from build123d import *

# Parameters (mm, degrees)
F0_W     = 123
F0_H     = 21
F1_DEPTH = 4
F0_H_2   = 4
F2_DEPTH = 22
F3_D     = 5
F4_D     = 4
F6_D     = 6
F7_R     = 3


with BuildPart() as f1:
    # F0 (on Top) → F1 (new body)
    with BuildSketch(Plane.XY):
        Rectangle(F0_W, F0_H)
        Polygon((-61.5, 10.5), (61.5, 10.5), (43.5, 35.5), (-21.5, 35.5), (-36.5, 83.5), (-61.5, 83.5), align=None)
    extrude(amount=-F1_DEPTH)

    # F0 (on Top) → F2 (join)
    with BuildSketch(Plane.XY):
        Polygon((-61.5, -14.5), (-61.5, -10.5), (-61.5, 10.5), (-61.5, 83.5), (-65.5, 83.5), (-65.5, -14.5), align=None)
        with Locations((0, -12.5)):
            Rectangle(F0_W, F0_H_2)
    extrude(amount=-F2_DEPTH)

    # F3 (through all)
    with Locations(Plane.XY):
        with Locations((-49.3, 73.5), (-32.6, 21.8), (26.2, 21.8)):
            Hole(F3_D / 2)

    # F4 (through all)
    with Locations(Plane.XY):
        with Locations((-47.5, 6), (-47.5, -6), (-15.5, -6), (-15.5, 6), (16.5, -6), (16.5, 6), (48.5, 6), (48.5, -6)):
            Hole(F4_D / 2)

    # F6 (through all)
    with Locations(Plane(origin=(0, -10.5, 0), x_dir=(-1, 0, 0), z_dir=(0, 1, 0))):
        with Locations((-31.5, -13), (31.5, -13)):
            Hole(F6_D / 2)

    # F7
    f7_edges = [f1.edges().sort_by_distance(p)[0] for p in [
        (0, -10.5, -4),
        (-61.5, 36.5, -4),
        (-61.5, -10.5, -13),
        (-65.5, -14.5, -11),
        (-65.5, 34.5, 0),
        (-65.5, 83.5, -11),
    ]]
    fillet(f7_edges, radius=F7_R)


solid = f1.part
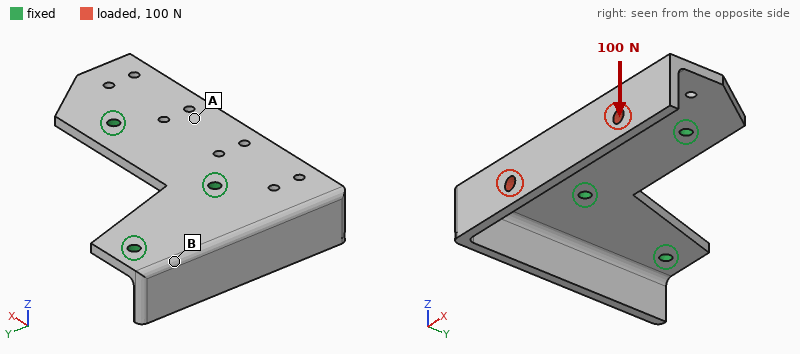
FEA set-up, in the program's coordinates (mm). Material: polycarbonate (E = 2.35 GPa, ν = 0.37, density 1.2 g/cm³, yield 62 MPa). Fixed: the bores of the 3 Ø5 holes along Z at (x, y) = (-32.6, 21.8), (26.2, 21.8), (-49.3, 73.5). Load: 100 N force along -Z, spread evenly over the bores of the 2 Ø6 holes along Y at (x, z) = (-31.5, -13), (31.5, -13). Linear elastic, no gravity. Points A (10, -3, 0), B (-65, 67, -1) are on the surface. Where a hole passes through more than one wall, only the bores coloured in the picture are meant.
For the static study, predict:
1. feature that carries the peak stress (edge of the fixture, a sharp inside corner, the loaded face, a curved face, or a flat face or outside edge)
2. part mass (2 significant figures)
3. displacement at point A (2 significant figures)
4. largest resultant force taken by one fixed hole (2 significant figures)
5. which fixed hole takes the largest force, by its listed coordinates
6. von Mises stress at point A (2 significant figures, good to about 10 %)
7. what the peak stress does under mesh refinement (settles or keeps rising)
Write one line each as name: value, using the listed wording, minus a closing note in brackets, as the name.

feature that carries the peak stress: edge of the fixture
part mass: 56 g
displacement at point A: 0.62 mm
largest resultant force taken by one fixed hole: 71 N
which fixed hole takes the largest force, by its listed coordinates: (-32.6, 21.8)
von Mises stress at point A: 3.3 MPa
what the peak stress does under mesh refinement: keeps rising
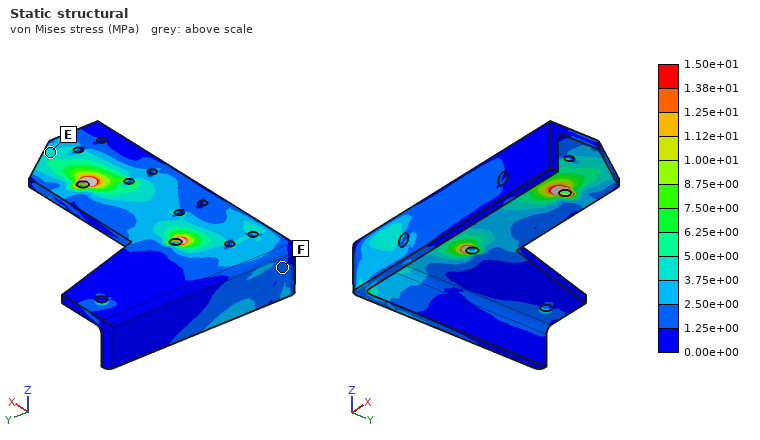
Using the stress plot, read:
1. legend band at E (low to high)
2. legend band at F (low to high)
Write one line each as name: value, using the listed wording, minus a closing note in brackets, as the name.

legend band at E: 3.75e+00 to 5.00e+00 MPa
legend band at F: 1.25e+00 to 2.50e+00 MPa
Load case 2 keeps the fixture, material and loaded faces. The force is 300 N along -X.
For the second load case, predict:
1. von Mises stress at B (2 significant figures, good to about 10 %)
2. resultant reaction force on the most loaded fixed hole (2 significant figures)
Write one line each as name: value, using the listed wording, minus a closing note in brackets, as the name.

von Mises stress at B: 1.3 MPa
resultant reaction force on the most loaded fixed hole: 210 N
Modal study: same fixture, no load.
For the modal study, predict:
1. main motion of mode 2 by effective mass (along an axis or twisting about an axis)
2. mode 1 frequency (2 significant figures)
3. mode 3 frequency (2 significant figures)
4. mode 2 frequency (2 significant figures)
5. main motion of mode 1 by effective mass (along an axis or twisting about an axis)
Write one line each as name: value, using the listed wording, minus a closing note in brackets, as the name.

main motion of mode 2 by effective mass: along Z
mode 1 frequency: 350 Hz
mode 3 frequency: 1000 Hz
mode 2 frequency: 420 Hz
main motion of mode 1 by effective mass: along Z
